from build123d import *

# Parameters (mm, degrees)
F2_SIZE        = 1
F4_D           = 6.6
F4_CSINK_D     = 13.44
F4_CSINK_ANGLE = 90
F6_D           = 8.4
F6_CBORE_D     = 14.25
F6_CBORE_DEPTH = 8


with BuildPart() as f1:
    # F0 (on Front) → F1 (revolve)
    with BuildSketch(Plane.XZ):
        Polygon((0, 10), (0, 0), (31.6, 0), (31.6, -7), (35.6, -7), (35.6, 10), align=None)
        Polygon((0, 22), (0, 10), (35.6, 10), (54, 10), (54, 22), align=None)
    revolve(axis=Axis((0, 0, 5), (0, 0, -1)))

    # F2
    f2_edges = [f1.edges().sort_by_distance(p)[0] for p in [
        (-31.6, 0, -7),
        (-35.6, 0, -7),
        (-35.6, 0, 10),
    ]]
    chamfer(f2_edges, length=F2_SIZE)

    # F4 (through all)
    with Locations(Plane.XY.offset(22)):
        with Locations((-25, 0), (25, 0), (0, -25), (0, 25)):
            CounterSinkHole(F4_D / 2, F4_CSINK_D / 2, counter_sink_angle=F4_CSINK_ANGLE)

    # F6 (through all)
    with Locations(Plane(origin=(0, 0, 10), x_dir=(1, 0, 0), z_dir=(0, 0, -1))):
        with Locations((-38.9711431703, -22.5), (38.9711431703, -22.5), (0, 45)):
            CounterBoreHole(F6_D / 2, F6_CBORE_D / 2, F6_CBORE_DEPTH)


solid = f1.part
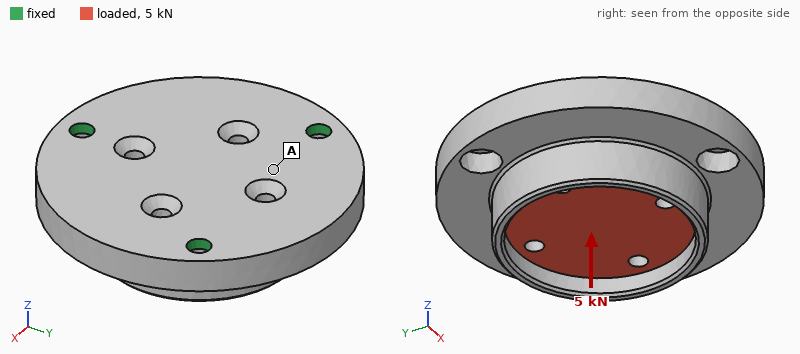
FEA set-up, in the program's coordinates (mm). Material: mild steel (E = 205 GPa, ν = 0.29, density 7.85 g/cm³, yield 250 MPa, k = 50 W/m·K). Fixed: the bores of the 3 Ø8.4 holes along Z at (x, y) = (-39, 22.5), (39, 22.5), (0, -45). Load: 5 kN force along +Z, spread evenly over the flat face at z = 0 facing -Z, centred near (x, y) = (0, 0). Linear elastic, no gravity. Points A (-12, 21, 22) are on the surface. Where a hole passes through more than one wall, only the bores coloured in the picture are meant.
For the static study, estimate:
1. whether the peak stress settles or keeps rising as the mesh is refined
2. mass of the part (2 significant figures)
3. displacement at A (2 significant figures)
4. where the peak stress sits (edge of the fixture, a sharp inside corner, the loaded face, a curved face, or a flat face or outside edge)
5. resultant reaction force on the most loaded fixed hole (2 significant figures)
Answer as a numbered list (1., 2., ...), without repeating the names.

1. keeps rising
2. 1.2 kg
3. 3.3 µm
4. edge of the fixture
5. 2.1 kN
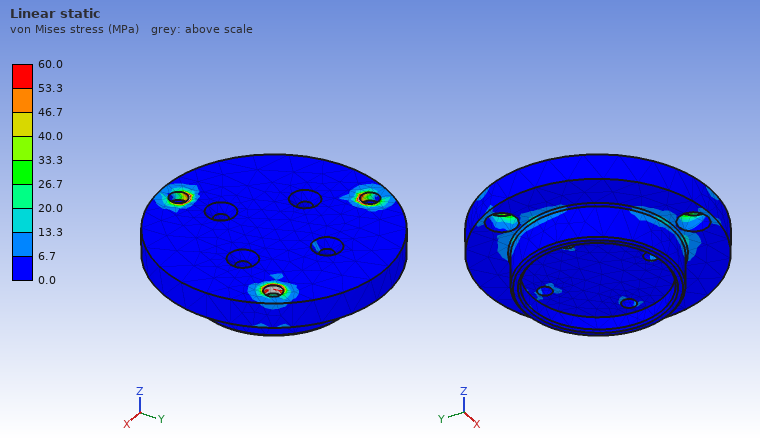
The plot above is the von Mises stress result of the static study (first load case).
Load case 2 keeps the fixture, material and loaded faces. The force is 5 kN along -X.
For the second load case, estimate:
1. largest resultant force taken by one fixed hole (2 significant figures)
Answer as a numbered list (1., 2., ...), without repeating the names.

1. 2.4 kN
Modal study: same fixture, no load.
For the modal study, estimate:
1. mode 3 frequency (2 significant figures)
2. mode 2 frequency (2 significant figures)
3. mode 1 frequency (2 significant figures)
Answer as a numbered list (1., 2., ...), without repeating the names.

1. 6200 Hz
2. 6100 Hz
3. 6100 Hz
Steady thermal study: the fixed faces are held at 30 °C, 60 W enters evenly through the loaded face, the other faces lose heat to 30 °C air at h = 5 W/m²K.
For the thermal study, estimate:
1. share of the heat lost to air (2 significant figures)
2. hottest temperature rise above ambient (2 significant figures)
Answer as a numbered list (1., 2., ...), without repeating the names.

1. 4.6 %
2. 32 K
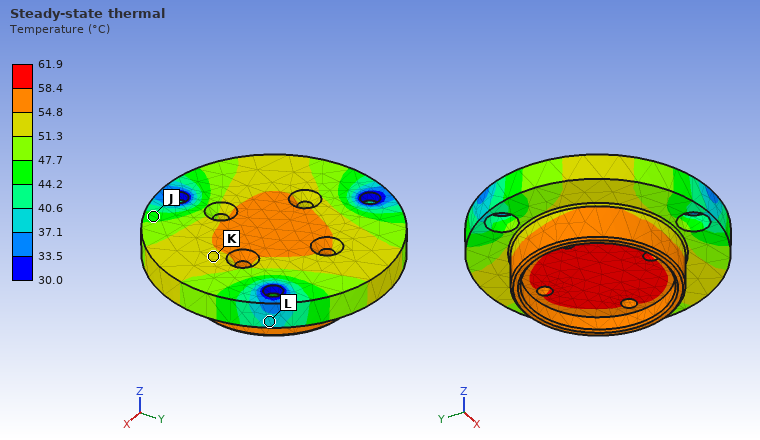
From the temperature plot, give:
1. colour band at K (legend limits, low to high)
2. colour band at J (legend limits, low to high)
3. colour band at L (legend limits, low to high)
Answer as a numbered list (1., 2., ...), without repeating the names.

1. 51.3 to 54.8 °C
2. 44.2 to 47.7 °C
3. 37.1 to 40.6 °C
